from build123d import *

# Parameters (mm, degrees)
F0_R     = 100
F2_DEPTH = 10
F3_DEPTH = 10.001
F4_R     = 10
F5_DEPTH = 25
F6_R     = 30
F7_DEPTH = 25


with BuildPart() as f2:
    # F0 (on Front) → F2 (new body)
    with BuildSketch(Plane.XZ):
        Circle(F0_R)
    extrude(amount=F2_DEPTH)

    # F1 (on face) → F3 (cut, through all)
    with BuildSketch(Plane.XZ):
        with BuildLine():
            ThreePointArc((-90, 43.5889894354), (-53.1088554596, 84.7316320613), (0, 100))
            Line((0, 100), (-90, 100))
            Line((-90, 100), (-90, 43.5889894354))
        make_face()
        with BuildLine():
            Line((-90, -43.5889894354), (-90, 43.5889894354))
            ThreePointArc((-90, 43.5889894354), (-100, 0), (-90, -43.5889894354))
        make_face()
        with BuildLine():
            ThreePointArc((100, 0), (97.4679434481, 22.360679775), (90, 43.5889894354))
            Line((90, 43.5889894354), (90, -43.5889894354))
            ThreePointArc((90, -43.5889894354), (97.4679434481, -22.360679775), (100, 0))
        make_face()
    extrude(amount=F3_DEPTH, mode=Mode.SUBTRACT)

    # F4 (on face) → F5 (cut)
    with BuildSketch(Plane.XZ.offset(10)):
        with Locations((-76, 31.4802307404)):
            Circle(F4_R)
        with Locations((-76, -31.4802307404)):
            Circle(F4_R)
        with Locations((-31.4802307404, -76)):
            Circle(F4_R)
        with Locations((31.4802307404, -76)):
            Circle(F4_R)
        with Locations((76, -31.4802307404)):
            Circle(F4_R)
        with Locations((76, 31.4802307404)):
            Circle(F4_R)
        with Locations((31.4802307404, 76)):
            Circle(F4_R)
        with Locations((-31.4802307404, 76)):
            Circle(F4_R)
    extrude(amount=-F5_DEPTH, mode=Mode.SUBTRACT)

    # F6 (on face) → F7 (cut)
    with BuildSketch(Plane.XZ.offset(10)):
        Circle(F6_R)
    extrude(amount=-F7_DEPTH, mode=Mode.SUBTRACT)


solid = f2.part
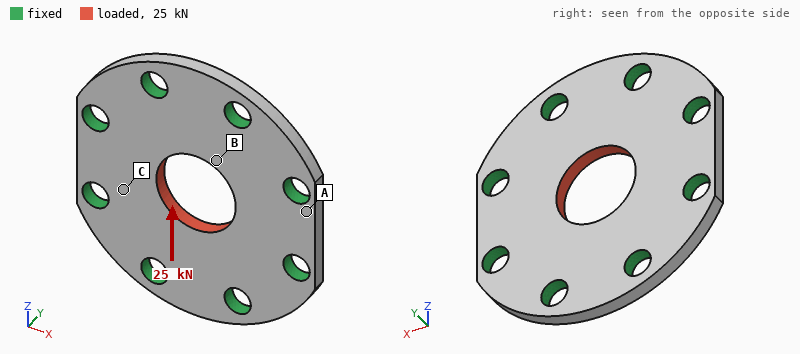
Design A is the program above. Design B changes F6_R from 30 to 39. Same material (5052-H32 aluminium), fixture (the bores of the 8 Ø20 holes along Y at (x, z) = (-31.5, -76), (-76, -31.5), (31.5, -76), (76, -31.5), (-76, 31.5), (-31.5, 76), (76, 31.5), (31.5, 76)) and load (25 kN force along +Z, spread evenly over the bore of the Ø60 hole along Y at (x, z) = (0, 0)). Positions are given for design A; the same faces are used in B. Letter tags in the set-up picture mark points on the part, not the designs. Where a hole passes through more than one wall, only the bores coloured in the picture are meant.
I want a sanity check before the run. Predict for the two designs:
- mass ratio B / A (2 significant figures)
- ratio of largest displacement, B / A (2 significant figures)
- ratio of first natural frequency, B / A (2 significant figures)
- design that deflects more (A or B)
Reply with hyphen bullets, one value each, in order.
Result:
- 0.92
- 0.75
- 1.3
- A
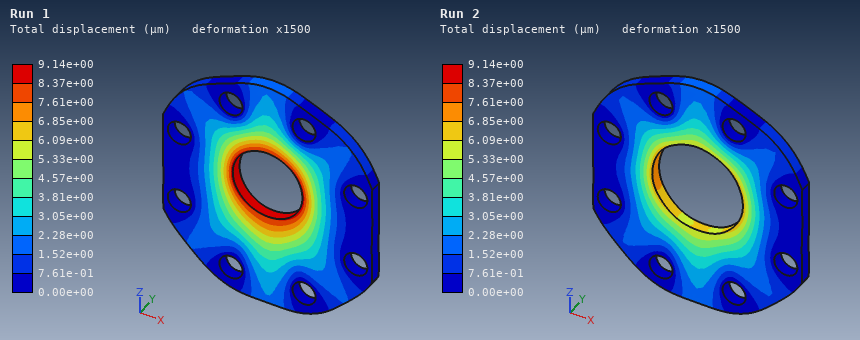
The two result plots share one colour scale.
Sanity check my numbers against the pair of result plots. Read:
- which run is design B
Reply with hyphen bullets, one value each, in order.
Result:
- Run 2
